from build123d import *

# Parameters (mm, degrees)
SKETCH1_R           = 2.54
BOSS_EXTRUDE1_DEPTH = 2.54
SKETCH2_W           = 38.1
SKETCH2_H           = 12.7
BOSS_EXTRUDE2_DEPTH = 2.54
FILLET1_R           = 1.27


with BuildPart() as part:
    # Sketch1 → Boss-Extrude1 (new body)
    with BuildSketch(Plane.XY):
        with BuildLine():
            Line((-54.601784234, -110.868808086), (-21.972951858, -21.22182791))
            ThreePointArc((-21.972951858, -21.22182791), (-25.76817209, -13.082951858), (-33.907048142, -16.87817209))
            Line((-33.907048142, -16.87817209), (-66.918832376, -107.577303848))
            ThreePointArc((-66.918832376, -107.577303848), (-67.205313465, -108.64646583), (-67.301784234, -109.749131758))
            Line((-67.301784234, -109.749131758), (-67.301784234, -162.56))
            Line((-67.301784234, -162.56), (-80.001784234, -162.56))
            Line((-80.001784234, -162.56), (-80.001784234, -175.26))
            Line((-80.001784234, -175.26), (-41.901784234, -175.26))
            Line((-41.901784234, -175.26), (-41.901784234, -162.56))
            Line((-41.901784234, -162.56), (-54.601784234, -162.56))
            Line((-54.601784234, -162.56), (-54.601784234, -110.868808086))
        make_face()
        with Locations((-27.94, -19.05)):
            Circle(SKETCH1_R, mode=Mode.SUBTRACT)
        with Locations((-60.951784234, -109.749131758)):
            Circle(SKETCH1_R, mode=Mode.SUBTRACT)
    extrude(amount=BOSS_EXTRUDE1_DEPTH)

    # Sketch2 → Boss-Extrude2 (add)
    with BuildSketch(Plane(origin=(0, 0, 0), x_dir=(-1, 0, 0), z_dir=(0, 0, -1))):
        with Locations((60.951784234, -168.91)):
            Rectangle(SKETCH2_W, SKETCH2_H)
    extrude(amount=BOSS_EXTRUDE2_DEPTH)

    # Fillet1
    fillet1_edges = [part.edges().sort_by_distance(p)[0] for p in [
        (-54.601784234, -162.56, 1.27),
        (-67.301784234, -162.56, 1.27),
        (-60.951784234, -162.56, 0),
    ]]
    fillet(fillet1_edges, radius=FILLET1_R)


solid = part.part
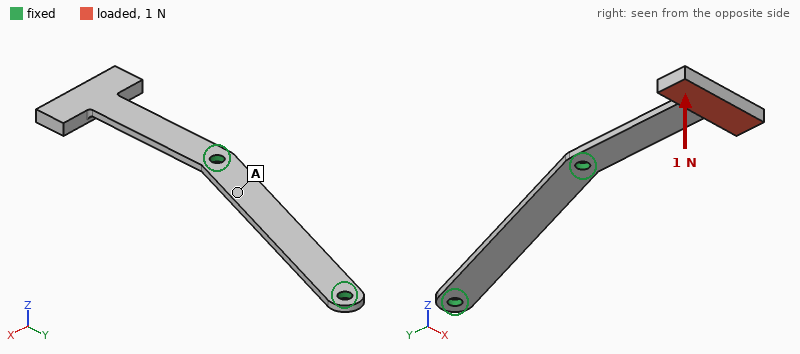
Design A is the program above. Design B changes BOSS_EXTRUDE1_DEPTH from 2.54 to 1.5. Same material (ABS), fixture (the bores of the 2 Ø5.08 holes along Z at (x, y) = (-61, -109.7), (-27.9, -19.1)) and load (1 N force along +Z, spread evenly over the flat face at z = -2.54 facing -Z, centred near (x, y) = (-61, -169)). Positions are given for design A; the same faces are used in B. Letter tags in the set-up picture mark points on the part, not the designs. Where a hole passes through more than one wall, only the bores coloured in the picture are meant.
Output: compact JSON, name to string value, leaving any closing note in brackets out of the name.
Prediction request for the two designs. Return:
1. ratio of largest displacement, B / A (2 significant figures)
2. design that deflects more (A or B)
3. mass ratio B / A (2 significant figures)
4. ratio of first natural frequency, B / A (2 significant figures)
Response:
{"ratio of largest displacement, B / A": "4.8", "design that deflects more": "B", "mass ratio B / A": "0.66", "ratio of first natural frequency, B / A": "0.52"}
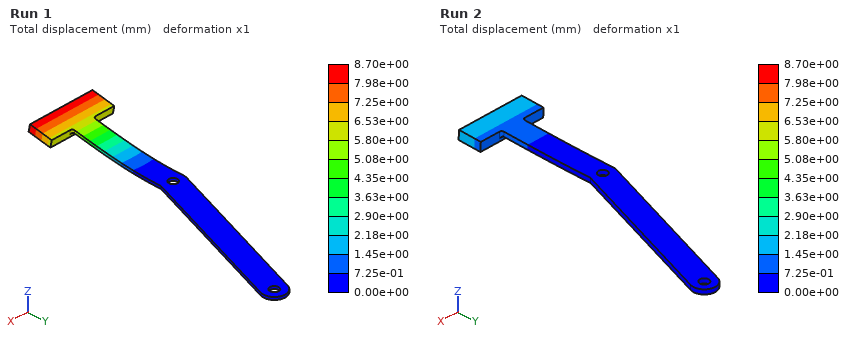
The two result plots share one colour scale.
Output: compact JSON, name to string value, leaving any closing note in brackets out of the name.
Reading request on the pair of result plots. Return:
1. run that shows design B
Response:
{"run that shows design B": "Run 1"}
